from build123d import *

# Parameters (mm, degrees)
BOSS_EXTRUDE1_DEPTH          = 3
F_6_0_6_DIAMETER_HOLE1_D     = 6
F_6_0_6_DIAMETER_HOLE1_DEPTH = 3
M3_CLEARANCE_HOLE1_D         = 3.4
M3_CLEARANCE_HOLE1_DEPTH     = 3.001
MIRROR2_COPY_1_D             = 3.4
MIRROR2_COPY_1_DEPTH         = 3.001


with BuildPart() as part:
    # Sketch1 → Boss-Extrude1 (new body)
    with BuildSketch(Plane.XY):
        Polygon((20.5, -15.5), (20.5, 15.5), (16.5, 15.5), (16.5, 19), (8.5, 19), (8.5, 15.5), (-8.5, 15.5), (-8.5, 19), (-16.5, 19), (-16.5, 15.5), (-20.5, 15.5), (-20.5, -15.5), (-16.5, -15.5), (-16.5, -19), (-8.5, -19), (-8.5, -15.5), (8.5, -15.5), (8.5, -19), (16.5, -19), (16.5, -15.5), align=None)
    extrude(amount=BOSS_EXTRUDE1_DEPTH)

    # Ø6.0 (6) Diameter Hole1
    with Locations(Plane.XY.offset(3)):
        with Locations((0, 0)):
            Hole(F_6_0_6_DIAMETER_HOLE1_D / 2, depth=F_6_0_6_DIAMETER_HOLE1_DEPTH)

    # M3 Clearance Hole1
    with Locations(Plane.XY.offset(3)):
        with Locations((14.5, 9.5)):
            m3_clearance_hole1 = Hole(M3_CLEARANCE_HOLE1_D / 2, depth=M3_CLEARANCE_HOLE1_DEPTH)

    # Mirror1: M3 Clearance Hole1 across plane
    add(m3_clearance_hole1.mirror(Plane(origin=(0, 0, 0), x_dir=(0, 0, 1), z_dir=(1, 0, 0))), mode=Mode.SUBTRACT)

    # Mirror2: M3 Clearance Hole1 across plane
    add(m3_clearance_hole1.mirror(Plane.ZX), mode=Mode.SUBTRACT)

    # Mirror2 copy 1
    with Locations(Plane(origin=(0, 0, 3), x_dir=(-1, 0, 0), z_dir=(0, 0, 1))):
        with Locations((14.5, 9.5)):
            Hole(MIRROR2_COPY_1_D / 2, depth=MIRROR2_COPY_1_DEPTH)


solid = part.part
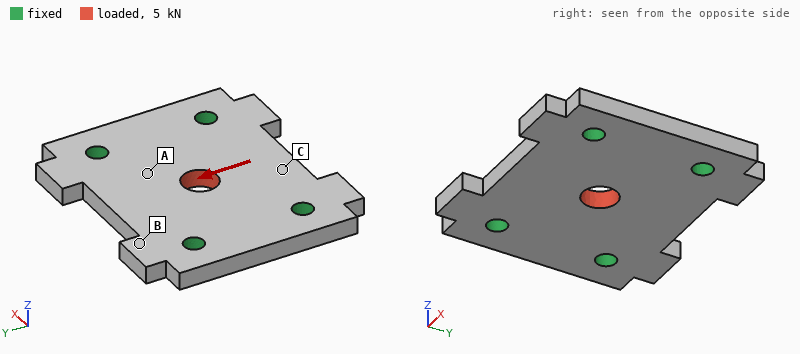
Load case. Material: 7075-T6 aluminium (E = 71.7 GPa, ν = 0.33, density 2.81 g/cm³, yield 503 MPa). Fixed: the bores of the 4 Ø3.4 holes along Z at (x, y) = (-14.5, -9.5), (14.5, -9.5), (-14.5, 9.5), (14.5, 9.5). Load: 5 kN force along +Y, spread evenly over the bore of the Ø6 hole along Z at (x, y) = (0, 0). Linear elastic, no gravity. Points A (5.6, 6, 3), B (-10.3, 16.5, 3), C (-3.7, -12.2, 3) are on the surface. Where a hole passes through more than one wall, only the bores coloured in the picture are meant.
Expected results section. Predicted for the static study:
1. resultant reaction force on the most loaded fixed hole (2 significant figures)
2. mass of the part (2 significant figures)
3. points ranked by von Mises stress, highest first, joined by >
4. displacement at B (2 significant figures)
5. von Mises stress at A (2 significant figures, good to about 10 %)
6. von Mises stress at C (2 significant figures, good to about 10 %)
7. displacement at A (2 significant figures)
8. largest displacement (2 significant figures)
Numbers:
1.4 kN
11 g
A > C > B
7.3 µm
60 MPa
30 MPa
11 µm
19 µm
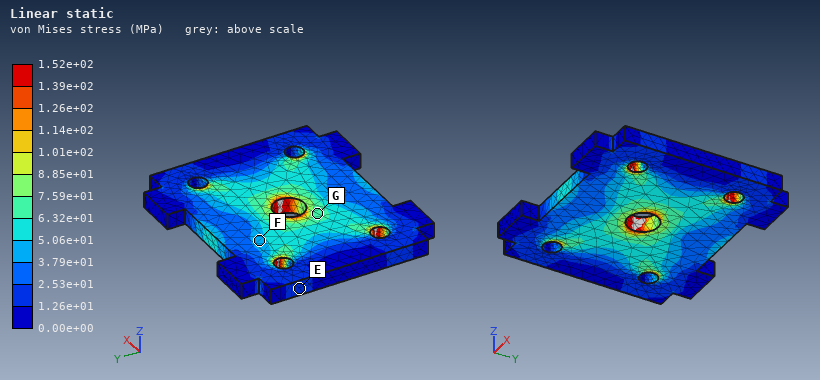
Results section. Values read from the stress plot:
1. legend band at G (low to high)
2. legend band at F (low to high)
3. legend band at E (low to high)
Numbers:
6.32e+01 to 7.59e+01 MPa
3.79e+01 to 5.06e+01 MPa
1.26e+01 to 2.53e+01 MPa
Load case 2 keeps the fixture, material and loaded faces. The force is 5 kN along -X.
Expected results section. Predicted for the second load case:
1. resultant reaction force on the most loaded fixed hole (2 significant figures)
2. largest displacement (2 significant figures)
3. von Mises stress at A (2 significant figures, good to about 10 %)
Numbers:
1.3 kN
12 µm
47 MPa
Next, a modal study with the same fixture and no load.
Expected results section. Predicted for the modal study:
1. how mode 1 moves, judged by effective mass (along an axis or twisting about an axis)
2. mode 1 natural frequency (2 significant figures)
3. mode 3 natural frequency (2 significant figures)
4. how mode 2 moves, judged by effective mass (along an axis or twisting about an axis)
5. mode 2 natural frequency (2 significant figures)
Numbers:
along Z
18 kHz
25 kHz
twisting about X
20 kHz
